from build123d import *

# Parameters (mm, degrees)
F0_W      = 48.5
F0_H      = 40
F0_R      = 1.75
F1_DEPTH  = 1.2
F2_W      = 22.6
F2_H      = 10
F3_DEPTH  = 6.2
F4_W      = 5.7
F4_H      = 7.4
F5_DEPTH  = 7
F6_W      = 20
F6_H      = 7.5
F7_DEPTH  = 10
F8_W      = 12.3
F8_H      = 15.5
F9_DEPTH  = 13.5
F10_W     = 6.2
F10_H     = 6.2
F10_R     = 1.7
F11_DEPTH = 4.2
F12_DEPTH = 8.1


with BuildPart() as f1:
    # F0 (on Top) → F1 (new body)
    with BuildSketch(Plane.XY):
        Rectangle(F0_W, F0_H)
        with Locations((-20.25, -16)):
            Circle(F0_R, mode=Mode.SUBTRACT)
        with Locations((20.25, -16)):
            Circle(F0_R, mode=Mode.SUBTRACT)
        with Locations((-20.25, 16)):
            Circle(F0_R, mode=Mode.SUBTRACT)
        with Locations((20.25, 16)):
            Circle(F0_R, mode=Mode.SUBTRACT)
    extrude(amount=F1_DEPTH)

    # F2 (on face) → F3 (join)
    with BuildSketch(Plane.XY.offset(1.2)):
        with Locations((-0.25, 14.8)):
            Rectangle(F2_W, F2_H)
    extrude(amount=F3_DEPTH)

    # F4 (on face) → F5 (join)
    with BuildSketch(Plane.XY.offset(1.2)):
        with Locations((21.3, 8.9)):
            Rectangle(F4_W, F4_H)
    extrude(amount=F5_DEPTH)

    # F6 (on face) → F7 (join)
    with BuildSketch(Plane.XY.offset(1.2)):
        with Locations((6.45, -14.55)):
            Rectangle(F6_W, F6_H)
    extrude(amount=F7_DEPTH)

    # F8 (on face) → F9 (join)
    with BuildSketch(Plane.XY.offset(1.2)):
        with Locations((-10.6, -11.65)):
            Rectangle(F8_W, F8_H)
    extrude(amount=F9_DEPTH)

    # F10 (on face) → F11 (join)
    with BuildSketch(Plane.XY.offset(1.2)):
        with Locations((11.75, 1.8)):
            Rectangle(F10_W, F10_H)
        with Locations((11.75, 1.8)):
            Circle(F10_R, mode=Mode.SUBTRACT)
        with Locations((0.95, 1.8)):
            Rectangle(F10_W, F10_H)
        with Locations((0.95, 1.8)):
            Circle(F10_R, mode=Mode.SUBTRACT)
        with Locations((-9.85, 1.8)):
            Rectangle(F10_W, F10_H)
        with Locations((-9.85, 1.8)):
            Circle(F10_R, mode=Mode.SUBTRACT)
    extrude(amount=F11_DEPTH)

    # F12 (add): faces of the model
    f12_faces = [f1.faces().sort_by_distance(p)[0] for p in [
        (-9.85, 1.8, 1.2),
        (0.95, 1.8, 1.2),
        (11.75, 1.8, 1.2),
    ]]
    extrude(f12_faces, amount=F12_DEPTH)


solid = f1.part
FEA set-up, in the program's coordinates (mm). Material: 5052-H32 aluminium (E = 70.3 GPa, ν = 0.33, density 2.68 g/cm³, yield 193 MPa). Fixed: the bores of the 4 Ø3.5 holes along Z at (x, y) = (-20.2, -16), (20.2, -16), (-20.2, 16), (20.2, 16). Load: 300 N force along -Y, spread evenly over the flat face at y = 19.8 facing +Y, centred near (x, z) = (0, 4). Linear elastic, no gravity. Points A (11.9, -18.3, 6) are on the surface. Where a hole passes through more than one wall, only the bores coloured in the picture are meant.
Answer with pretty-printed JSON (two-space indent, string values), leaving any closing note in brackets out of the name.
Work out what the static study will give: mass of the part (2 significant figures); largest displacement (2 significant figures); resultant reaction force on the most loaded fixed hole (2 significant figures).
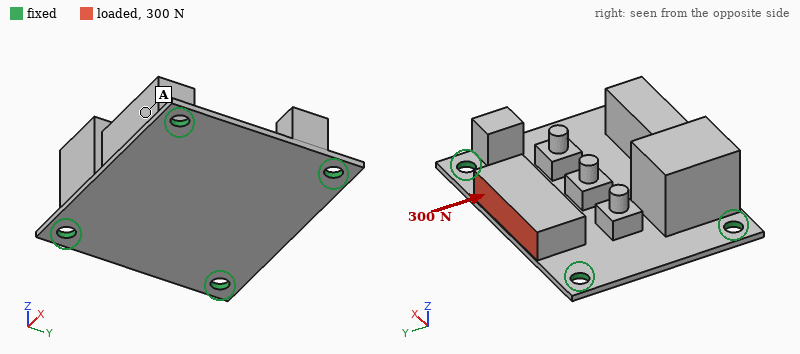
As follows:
{
  "mass of the part": "23 g",
  "largest displacement": "60 µm",
  "resultant reaction force on the most loaded fixed hole": "95 N"
}
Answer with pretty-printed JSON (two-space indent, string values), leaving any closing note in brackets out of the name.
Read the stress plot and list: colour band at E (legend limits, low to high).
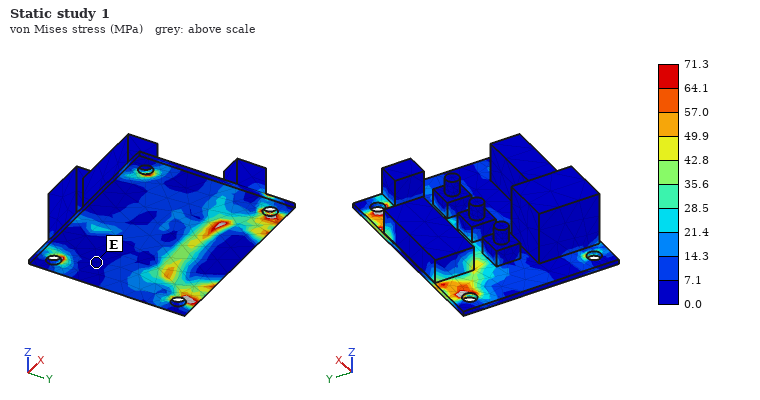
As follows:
{
  "colour band at E": "0.0 to 7.1 MPa"
}
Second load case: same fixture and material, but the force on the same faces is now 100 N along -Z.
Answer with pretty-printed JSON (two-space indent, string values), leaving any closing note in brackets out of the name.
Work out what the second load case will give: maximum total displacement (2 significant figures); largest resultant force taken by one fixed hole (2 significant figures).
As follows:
{
  "maximum total displacement": "49 µm",
  "largest resultant force taken by one fixed hole": "73 N"
}
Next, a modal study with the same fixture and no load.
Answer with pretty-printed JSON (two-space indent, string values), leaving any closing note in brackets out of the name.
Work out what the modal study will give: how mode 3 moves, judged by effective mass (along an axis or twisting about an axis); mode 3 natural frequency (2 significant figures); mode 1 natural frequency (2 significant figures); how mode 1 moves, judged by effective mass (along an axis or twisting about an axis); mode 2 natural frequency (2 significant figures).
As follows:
{
  "how mode 3 moves, judged by effective mass": "along Z",
  "mode 3 natural frequency": "5000 Hz",
  "mode 1 natural frequency": "2500 Hz",
  "how mode 1 moves, judged by effective mass": "along Z",
  "mode 2 natural frequency": "3300 Hz"
}
